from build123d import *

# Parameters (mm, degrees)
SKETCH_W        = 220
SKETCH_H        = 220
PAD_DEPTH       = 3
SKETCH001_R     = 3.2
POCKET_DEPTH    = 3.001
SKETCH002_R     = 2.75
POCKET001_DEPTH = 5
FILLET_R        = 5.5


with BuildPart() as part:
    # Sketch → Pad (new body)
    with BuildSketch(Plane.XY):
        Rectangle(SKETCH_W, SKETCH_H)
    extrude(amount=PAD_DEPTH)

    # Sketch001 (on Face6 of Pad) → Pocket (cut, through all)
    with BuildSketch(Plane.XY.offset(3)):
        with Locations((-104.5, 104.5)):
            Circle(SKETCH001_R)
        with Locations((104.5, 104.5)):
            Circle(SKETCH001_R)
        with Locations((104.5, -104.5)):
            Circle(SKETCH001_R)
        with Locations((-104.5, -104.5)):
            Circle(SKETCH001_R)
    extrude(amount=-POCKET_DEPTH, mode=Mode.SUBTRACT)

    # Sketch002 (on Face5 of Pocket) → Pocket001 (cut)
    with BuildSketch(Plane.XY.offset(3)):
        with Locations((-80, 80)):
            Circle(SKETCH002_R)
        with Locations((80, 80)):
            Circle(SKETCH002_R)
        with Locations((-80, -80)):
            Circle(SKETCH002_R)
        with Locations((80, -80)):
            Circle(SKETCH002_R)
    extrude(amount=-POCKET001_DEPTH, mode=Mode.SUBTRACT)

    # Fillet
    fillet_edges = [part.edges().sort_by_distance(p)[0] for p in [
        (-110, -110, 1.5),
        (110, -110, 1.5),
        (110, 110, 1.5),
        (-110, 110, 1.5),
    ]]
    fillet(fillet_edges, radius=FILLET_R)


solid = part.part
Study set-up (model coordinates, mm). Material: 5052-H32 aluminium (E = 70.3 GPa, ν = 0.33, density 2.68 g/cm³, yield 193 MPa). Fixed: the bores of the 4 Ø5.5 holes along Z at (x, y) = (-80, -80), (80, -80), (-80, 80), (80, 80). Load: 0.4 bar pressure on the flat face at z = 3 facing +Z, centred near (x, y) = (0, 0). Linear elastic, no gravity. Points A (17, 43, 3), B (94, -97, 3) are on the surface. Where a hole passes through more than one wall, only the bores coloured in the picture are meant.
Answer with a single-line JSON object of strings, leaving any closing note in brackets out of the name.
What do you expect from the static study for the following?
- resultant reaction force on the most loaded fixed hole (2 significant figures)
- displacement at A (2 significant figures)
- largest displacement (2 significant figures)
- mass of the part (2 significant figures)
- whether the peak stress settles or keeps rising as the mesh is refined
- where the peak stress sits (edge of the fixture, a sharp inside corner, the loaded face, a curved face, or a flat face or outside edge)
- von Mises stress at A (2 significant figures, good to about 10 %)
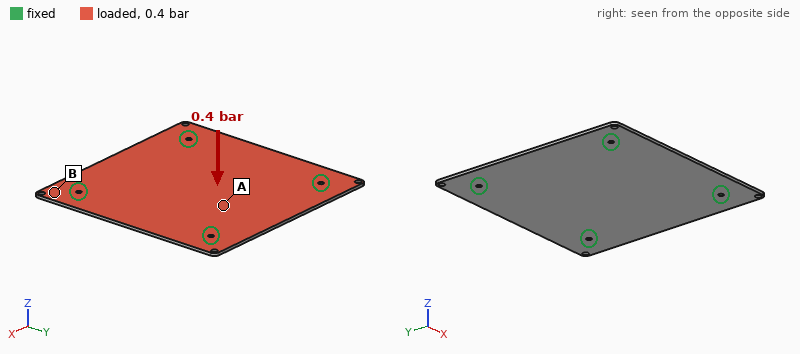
{"resultant reaction force on the most loaded fixed hole": "480 N", "displacement at A": "0.87 mm", "largest displacement": "1.1 mm", "mass of the part": "390 g", "whether the peak stress settles or keeps rising as the mesh is refined": "keeps rising", "where the peak stress sits": "edge of the fixture", "von Mises stress at A": "29 MPa"}
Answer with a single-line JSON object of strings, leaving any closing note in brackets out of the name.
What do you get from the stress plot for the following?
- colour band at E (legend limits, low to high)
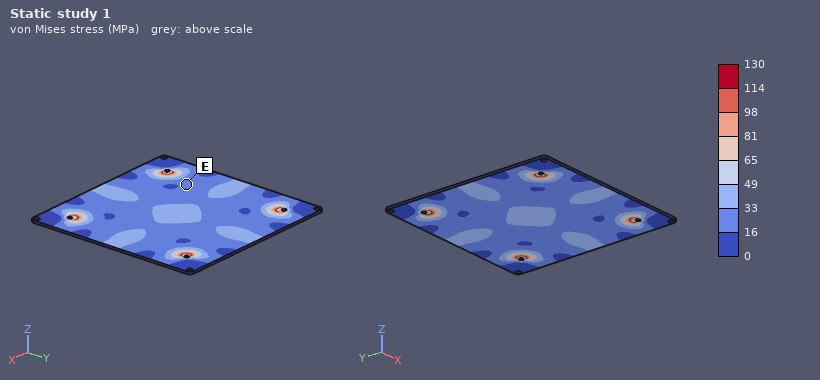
{"colour band at E": "16 to 33 MPa"}
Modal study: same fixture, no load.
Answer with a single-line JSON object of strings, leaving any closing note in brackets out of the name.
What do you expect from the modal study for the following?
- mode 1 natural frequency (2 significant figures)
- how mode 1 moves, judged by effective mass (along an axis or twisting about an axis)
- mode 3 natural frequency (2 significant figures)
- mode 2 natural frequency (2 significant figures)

{"mode 1 natural frequency": "410 Hz", "how mode 1 moves, judged by effective mass": "along Z", "mode 3 natural frequency": "630 Hz", "mode 2 natural frequency": "620 Hz"}
